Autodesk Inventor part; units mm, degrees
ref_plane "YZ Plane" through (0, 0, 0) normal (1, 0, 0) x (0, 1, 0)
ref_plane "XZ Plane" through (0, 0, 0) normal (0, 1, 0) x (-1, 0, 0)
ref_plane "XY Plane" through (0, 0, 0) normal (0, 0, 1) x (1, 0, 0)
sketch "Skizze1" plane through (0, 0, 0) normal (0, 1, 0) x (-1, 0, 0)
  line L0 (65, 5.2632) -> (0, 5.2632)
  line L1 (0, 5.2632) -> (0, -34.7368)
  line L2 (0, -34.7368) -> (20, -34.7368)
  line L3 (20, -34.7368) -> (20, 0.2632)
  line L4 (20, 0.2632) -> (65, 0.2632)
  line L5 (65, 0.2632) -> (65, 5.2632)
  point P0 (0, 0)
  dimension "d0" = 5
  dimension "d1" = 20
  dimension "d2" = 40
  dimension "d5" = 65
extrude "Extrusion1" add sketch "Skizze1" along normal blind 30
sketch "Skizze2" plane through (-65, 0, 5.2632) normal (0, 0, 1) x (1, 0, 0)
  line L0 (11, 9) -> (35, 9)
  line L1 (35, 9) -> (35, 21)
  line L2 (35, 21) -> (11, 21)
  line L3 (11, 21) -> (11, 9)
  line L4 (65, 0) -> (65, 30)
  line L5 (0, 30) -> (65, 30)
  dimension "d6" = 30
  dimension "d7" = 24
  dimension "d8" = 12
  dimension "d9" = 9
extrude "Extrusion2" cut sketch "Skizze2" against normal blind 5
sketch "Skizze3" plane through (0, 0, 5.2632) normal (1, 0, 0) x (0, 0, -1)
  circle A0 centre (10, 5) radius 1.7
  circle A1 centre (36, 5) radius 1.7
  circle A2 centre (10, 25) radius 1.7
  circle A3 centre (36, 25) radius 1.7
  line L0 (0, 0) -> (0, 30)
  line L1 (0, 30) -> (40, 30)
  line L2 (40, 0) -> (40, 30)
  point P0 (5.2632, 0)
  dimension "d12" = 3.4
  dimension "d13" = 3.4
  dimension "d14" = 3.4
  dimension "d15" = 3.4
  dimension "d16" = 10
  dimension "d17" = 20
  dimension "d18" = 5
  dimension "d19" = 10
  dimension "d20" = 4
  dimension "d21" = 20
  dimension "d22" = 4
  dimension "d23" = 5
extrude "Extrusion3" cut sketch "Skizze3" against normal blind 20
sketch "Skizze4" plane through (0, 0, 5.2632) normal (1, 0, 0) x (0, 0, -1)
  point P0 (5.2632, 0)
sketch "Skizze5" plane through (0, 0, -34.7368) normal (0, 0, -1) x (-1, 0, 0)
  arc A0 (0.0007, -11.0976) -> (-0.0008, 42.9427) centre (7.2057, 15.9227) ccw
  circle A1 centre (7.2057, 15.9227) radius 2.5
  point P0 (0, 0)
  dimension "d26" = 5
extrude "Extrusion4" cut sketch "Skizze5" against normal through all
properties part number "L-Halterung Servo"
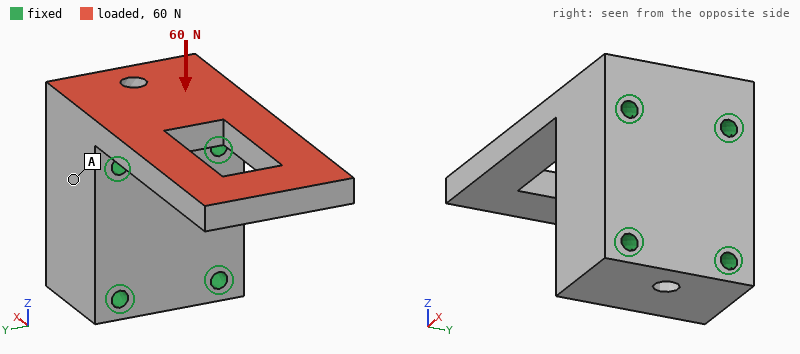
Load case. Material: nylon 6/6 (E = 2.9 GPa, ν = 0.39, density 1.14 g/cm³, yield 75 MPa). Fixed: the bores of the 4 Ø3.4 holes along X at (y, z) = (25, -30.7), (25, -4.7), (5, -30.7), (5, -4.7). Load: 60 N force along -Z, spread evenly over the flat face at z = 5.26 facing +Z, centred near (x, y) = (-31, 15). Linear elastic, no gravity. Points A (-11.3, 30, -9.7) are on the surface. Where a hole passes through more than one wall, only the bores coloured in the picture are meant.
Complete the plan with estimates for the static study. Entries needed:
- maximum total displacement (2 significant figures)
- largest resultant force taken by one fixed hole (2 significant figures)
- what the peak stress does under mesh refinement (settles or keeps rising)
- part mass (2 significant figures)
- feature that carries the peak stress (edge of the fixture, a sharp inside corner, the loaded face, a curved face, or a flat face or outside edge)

0.81 mm
29 N
keeps rising
32 g
a sharp inside corner
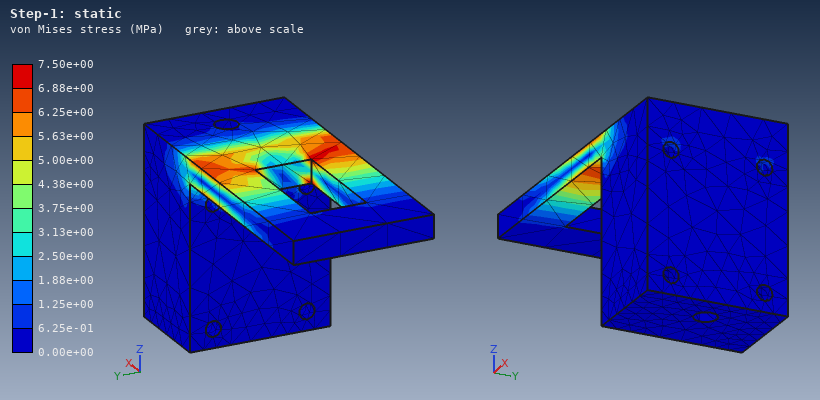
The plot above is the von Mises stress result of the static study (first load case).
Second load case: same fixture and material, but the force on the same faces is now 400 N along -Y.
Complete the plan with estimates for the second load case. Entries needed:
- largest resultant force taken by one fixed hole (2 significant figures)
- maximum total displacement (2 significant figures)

380 N
0.55 mm
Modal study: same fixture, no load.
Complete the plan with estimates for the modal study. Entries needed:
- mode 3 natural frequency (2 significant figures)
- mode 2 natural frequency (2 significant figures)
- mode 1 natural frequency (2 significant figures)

1700 Hz
1500 Hz
540 Hz
